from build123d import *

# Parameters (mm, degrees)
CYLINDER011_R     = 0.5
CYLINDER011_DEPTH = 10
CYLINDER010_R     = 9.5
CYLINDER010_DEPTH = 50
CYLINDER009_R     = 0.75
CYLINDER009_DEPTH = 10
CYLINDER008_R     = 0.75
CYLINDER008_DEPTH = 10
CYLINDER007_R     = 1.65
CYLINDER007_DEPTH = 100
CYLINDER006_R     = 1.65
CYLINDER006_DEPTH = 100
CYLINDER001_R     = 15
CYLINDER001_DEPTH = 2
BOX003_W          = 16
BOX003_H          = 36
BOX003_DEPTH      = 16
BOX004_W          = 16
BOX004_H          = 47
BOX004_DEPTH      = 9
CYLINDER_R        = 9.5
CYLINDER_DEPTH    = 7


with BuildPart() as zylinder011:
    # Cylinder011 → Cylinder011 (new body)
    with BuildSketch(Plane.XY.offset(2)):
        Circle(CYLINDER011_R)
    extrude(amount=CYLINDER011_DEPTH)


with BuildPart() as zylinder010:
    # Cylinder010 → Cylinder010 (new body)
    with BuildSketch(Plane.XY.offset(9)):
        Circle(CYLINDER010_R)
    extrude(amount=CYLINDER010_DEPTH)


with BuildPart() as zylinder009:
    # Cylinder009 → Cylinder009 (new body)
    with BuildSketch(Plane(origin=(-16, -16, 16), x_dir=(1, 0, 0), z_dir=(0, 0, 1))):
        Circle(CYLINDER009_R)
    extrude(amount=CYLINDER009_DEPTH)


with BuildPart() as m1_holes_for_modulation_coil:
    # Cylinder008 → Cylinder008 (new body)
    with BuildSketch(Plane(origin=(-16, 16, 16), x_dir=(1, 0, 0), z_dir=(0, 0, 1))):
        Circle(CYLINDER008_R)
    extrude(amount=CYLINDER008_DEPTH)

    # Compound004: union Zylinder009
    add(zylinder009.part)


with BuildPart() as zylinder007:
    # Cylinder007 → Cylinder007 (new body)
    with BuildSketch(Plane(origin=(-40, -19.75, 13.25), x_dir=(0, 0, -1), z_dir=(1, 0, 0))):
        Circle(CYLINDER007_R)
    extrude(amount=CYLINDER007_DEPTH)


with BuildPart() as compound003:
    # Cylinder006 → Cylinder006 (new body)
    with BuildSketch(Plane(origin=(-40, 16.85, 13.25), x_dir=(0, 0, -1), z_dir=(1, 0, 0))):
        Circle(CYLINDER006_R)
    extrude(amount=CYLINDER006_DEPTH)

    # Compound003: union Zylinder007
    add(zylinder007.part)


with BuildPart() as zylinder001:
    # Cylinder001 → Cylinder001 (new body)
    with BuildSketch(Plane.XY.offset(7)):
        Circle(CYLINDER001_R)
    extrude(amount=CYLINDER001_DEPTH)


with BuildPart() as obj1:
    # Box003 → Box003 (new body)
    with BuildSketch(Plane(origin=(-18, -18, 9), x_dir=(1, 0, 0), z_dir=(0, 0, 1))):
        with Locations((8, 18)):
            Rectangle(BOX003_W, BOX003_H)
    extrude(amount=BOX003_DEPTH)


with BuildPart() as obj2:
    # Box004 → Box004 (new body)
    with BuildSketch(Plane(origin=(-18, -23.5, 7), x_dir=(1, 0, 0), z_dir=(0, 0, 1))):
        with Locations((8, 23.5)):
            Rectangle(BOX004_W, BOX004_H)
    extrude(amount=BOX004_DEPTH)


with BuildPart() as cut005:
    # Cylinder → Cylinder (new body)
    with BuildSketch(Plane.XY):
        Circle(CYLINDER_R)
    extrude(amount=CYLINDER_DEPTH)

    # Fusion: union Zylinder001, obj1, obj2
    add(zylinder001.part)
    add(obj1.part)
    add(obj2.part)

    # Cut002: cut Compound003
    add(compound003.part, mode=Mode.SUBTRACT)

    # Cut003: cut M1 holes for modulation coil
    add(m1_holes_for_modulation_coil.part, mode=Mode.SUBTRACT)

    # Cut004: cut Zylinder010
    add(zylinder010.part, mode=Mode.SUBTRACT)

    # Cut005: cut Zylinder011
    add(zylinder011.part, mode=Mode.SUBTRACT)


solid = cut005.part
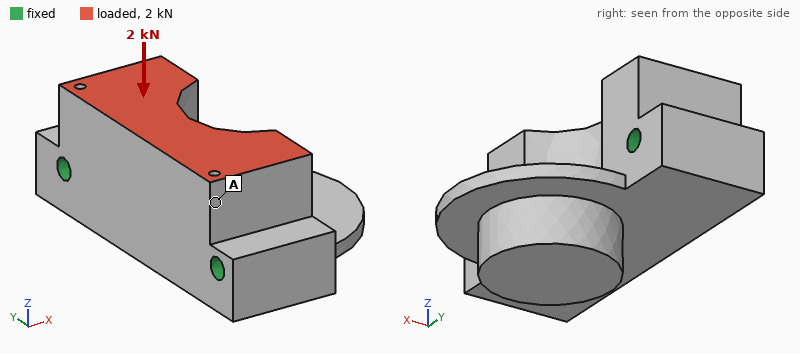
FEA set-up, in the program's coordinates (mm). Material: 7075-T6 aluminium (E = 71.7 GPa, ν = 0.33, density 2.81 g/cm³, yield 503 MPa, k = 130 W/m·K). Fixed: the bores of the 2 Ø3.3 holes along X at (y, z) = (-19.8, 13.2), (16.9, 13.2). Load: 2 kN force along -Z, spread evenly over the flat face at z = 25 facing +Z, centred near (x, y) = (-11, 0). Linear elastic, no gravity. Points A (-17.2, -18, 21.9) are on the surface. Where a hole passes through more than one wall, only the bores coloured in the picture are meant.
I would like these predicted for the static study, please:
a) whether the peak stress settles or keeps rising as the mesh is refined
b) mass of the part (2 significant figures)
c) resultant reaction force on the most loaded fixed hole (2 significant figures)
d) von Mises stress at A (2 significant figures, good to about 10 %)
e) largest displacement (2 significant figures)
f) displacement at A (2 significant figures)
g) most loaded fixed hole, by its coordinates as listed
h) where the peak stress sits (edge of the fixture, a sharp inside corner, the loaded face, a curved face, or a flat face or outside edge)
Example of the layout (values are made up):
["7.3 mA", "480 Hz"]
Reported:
["keeps rising", "36 g", "1.1 kN", "4.9 MPa", "4.2 µm", "1.7 µm", "(16.9, 13.2)", "edge of the fixture"]
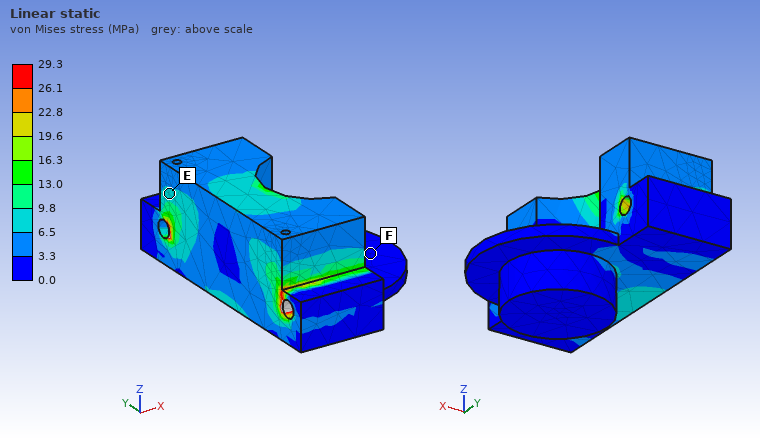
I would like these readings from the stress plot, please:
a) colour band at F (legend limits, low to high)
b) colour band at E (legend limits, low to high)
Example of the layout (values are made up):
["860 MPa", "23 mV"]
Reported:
["0.0 to 3.3 MPa", "6.5 to 9.8 MPa"]
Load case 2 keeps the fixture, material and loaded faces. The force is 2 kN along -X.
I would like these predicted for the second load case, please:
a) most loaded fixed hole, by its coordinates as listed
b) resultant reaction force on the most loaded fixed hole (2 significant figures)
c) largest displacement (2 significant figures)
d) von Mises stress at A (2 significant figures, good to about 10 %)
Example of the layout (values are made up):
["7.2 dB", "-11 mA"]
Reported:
["(16.9, 13.2)", "1.1 kN", "12 µm", "7.2 MPa"]
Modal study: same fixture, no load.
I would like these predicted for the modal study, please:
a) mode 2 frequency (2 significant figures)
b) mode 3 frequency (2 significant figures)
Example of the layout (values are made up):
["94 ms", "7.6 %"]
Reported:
["24 kHz", "24 kHz"]
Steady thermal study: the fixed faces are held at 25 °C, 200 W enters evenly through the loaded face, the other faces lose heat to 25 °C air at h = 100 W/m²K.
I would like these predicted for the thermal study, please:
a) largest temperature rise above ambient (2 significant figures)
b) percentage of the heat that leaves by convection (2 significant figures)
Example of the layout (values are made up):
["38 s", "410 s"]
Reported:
["61 K", "4.6 %"]
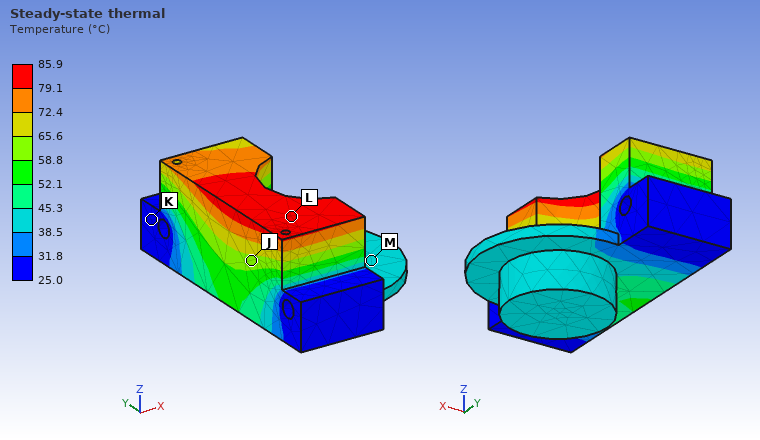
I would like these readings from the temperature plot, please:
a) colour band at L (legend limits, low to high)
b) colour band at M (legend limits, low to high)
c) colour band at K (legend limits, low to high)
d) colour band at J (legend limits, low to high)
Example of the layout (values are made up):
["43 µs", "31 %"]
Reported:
["79.1 to 85.9 °C", "38.5 to 45.3 °C", "25.0 to 31.8 °C", "58.8 to 65.6 °C"]
